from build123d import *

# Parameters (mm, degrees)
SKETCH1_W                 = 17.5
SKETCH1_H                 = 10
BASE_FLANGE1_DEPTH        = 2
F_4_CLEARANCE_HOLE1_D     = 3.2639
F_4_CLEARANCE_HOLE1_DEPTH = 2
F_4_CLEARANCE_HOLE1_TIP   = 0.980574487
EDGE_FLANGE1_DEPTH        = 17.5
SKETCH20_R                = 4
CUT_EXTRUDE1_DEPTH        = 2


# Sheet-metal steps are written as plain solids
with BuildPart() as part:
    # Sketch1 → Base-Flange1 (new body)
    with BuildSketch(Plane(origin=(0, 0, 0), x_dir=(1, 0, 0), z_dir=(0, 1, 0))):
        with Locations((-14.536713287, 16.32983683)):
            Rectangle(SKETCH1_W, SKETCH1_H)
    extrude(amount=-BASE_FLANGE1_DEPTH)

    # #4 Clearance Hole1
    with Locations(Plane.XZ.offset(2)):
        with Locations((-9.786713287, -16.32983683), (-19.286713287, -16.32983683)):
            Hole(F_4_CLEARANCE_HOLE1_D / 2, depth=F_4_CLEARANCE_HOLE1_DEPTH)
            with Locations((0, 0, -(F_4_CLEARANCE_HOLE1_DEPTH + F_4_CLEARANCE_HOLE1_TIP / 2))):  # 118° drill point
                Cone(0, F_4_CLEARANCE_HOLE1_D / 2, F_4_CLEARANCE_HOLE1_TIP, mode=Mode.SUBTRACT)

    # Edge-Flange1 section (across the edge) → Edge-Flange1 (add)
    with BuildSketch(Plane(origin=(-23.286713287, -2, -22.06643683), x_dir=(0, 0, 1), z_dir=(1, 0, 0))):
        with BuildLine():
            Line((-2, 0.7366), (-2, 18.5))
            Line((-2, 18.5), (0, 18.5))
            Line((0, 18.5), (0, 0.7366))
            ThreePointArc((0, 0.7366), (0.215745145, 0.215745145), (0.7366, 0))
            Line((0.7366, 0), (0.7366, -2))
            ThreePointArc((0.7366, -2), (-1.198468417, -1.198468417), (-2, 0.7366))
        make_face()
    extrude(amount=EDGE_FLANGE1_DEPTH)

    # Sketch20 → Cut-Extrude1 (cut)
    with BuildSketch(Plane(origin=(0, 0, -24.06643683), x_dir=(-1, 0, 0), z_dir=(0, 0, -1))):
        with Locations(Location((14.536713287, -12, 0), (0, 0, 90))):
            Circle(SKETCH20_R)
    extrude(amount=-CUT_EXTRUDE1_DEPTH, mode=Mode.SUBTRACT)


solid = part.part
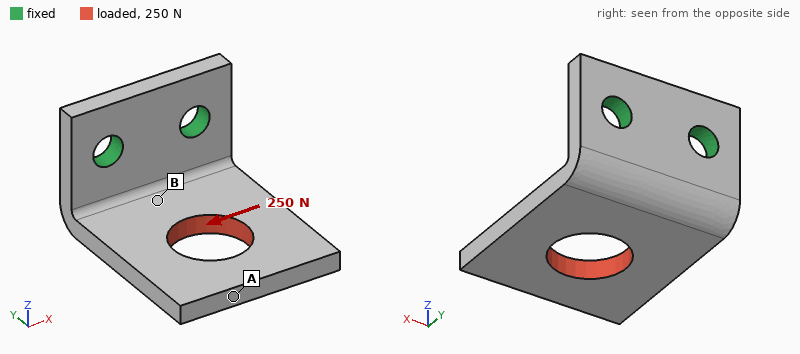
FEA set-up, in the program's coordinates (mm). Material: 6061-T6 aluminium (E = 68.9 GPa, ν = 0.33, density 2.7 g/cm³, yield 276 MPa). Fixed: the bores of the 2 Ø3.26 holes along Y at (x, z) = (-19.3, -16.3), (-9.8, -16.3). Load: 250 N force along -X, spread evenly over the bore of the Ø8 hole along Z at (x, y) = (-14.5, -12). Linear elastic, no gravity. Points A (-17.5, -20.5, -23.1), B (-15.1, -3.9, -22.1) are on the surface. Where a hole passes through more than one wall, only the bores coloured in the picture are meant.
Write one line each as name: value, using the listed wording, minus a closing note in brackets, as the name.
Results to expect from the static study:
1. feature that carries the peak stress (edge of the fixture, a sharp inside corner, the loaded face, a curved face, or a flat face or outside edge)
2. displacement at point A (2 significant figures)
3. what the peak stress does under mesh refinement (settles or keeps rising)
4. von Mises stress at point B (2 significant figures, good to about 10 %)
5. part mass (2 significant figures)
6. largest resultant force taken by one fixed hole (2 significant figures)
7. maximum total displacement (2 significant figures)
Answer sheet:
feature that carries the peak stress: edge of the fixture
displacement at point A: 0.090 mm
what the peak stress does under mesh refinement: keeps rising
von Mises stress at point B: 66 MPa
part mass: 2.5 g
largest resultant force taken by one fixed hole: 290 N
maximum total displacement: 0.10 mm
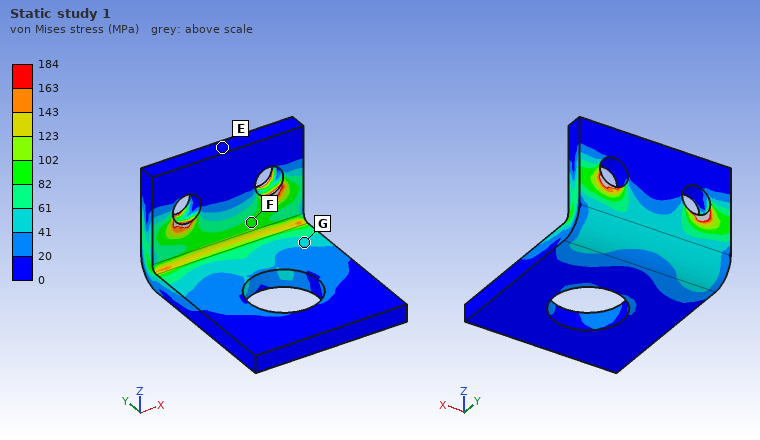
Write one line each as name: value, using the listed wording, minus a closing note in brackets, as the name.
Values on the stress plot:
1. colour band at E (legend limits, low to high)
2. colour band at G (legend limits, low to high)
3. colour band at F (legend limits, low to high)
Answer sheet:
colour band at E: 0 to 20 MPa
colour band at G: 41 to 61 MPa
colour band at F: 82 to 102 MPa
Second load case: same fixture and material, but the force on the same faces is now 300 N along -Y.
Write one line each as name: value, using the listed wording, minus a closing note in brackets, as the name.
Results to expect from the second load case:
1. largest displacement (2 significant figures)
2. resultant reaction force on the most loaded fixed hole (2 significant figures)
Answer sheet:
largest displacement: 0.12 mm
resultant reaction force on the most loaded fixed hole: 150 N
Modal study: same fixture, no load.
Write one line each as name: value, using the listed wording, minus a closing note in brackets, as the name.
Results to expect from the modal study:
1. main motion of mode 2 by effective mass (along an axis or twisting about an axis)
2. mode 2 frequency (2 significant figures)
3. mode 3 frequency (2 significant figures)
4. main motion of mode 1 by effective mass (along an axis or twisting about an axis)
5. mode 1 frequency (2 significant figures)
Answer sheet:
main motion of mode 2 by effective mass: along X
mode 2 frequency: 7200 Hz
mode 3 frequency: 10 kHz
main motion of mode 1 by effective mass: along Z
mode 1 frequency: 3100 Hz
